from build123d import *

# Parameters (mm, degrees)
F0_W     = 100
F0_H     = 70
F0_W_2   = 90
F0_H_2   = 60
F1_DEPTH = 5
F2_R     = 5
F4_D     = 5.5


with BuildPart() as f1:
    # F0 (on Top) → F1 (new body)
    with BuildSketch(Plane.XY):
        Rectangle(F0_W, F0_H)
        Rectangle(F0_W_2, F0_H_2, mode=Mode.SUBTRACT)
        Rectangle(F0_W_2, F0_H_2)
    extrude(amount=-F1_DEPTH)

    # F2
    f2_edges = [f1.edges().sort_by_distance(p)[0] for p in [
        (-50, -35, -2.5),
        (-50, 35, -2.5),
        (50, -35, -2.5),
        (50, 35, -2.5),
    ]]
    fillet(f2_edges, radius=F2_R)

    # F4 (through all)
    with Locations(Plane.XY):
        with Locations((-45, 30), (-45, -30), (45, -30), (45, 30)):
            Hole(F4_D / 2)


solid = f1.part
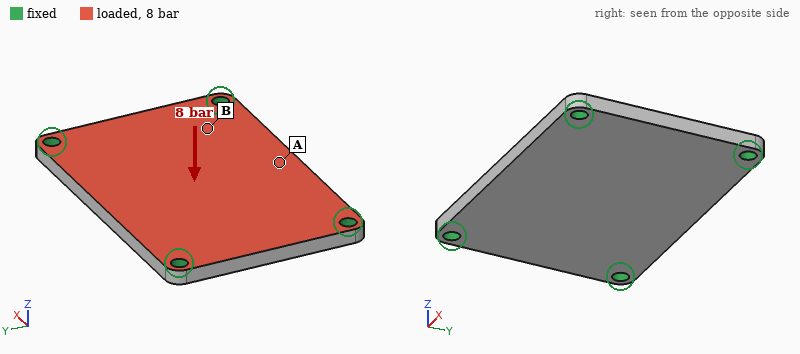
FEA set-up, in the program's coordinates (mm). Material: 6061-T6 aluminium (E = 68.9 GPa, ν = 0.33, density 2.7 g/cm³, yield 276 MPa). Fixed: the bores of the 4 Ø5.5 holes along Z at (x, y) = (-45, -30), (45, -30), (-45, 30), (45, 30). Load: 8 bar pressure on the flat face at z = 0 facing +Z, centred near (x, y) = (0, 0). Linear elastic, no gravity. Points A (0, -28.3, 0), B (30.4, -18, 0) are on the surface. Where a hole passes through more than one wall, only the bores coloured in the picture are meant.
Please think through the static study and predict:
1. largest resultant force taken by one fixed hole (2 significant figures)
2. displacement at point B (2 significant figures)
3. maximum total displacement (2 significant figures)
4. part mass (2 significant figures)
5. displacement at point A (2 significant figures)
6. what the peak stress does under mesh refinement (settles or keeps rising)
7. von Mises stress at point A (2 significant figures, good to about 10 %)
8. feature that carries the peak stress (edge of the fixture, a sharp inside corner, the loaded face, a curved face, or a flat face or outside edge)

1.4 kN
0.12 mm
0.29 mm
93 g
0.26 mm
keeps rising
79 MPa
edge of the fixture
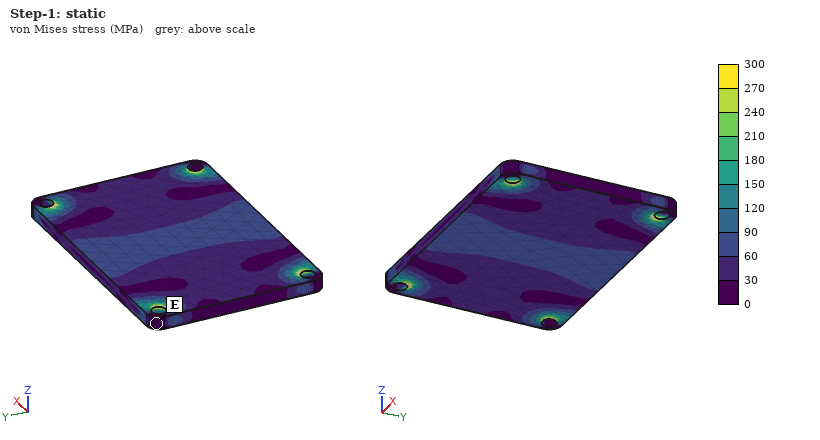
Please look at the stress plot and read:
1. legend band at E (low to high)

0 to 30 MPa
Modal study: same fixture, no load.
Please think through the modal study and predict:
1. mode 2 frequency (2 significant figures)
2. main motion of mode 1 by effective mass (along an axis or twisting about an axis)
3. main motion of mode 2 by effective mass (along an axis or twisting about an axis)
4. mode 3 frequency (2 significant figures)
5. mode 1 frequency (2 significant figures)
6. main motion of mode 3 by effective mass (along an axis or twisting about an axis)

4200 Hz
along Z
twisting about X
6400 Hz
2600 Hz
twisting about Y
